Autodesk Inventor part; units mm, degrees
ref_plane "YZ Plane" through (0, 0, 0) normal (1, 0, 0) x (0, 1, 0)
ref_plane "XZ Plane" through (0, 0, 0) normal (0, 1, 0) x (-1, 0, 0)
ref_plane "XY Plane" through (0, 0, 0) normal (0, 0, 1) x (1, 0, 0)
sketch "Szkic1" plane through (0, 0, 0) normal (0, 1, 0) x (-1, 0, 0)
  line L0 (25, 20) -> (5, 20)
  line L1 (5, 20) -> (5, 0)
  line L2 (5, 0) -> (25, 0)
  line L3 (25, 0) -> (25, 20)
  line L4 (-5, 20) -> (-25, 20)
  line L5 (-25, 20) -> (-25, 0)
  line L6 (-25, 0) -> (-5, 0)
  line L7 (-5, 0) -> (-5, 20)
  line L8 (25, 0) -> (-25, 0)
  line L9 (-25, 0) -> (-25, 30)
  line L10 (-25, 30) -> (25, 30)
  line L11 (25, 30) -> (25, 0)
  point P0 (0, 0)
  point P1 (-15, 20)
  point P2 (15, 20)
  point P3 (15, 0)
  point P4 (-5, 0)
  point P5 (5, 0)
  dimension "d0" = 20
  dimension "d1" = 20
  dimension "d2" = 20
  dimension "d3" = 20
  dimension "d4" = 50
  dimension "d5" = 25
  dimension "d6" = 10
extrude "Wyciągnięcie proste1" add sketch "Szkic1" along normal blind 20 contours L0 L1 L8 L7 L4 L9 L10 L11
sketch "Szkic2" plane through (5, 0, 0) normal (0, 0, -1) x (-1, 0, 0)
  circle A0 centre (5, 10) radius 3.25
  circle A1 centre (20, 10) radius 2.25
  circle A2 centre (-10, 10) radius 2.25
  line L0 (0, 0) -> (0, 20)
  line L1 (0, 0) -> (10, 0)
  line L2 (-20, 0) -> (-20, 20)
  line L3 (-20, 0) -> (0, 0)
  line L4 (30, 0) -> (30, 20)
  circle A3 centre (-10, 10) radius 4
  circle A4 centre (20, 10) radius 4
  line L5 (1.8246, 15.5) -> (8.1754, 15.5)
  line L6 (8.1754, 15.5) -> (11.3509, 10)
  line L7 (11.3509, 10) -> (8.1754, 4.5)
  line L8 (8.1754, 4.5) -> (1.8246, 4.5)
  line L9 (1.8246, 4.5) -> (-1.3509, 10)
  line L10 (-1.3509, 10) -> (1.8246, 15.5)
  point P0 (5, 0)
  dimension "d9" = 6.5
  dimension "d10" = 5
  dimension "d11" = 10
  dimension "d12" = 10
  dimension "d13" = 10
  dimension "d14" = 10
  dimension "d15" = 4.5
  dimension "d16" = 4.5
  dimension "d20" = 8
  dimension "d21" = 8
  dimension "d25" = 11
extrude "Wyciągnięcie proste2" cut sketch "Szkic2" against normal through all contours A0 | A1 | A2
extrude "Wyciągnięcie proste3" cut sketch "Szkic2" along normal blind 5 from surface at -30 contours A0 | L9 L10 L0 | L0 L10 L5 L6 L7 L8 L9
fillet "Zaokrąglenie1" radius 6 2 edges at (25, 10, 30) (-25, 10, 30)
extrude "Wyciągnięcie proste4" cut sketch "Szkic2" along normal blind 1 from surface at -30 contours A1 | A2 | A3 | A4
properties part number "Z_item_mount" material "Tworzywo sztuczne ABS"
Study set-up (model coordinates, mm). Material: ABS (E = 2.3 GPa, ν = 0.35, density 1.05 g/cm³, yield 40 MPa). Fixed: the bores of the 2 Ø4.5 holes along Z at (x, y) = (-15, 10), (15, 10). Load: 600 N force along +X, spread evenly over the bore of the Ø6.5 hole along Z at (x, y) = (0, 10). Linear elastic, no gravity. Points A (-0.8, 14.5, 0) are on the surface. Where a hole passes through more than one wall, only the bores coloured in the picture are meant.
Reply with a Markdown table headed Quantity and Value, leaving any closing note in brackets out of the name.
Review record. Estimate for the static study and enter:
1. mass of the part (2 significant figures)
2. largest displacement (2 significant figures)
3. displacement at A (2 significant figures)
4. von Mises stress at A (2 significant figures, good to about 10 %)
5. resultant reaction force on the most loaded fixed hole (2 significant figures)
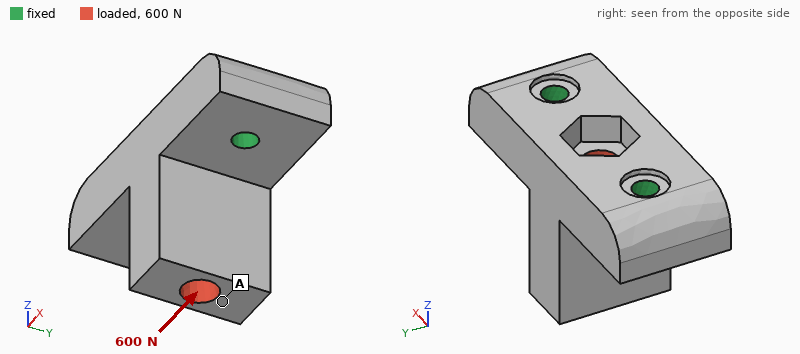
| Quantity | Value |
|---|---|
| mass of the part | 13 g |
| largest displacement | 0.37 mm |
| displacement at A | 0.35 mm |
| von Mises stress at A | 2.2 MPa |
| resultant reaction force on the most loaded fixed hole | 430 N |
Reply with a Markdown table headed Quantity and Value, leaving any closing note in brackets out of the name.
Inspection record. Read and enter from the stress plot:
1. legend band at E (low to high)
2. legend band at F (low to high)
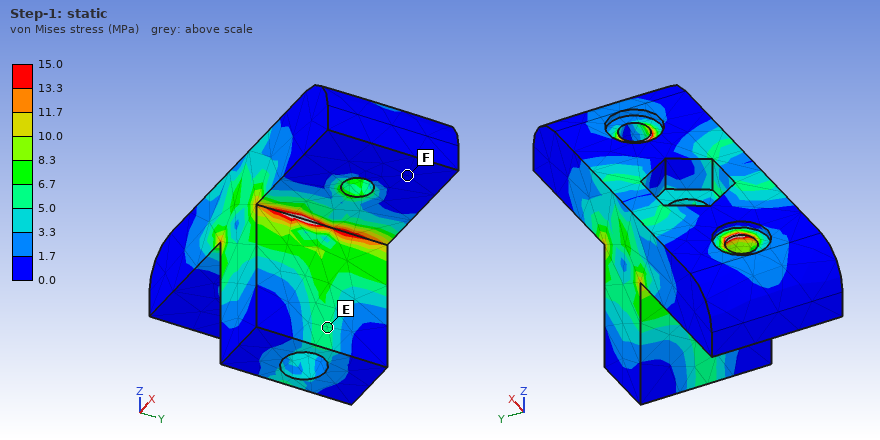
| Quantity | Value |
|---|---|
| legend band at E | 5.0 to 6.7 MPa |
| legend band at F | 0.0 to 1.7 MPa |
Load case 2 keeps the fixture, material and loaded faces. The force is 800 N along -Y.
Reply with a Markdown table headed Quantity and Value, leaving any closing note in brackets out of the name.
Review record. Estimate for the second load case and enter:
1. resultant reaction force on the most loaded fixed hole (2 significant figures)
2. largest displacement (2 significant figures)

| Quantity | Value |
|---|---|
| resultant reaction force on the most loaded fixed hole | 400 N |
| largest displacement | 0.62 mm |
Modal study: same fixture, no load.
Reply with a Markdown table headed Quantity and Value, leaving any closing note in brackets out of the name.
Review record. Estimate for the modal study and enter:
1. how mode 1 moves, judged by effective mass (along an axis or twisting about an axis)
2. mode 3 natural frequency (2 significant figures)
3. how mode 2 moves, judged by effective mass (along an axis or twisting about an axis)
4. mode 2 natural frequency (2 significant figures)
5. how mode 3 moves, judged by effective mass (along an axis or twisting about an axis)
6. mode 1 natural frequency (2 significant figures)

| Quantity | Value |
|---|---|
| how mode 1 moves, judged by effective mass | along Y |
| mode 3 natural frequency | 6700 Hz |
| how mode 2 moves, judged by effective mass | along X |
| mode 2 natural frequency | 3800 Hz |
| how mode 3 moves, judged by effective mass | along Z |
| mode 1 natural frequency | 3100 Hz |
